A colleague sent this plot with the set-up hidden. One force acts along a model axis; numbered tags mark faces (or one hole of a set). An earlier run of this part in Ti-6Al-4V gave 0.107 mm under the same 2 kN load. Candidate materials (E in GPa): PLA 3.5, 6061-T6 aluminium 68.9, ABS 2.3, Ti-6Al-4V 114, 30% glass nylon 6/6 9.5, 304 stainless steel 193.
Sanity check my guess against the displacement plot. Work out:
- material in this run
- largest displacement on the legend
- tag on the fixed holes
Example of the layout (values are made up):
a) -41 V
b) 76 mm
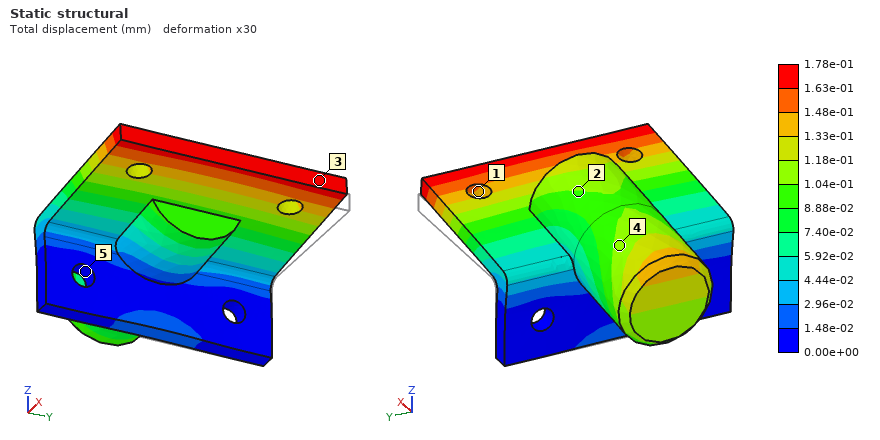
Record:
a) 6061-T6 aluminium
b) 1.78e-01 mm
c) 5
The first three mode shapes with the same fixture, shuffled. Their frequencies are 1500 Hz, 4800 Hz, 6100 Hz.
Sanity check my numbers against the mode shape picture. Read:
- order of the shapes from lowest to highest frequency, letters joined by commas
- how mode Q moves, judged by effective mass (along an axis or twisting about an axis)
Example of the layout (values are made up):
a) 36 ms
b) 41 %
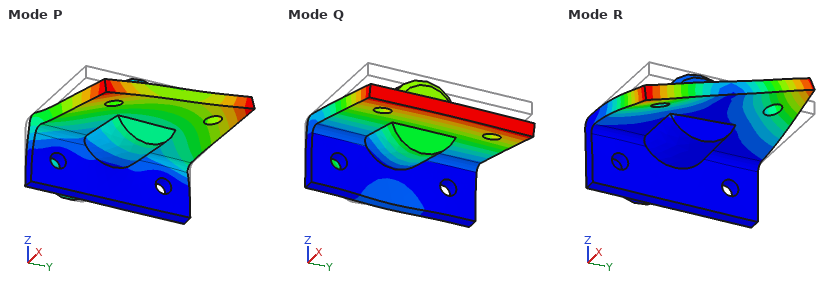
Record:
a) Q, P, R
b) along X
